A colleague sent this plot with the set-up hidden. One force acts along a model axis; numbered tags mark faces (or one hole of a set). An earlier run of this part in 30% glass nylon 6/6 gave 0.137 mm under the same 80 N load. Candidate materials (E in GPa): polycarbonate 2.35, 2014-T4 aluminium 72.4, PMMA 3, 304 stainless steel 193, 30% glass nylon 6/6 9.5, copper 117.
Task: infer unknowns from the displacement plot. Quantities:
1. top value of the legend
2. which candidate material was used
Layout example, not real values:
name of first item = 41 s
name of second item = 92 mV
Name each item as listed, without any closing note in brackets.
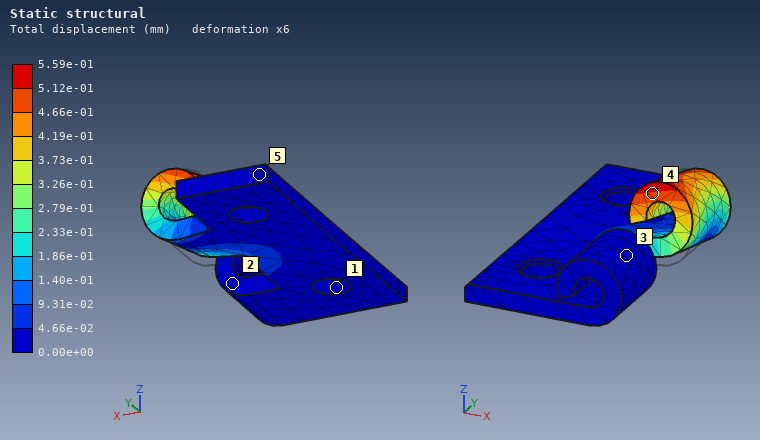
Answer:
top value of the legend = 5.59e-01 mm
which candidate material was used = polycarbonate
